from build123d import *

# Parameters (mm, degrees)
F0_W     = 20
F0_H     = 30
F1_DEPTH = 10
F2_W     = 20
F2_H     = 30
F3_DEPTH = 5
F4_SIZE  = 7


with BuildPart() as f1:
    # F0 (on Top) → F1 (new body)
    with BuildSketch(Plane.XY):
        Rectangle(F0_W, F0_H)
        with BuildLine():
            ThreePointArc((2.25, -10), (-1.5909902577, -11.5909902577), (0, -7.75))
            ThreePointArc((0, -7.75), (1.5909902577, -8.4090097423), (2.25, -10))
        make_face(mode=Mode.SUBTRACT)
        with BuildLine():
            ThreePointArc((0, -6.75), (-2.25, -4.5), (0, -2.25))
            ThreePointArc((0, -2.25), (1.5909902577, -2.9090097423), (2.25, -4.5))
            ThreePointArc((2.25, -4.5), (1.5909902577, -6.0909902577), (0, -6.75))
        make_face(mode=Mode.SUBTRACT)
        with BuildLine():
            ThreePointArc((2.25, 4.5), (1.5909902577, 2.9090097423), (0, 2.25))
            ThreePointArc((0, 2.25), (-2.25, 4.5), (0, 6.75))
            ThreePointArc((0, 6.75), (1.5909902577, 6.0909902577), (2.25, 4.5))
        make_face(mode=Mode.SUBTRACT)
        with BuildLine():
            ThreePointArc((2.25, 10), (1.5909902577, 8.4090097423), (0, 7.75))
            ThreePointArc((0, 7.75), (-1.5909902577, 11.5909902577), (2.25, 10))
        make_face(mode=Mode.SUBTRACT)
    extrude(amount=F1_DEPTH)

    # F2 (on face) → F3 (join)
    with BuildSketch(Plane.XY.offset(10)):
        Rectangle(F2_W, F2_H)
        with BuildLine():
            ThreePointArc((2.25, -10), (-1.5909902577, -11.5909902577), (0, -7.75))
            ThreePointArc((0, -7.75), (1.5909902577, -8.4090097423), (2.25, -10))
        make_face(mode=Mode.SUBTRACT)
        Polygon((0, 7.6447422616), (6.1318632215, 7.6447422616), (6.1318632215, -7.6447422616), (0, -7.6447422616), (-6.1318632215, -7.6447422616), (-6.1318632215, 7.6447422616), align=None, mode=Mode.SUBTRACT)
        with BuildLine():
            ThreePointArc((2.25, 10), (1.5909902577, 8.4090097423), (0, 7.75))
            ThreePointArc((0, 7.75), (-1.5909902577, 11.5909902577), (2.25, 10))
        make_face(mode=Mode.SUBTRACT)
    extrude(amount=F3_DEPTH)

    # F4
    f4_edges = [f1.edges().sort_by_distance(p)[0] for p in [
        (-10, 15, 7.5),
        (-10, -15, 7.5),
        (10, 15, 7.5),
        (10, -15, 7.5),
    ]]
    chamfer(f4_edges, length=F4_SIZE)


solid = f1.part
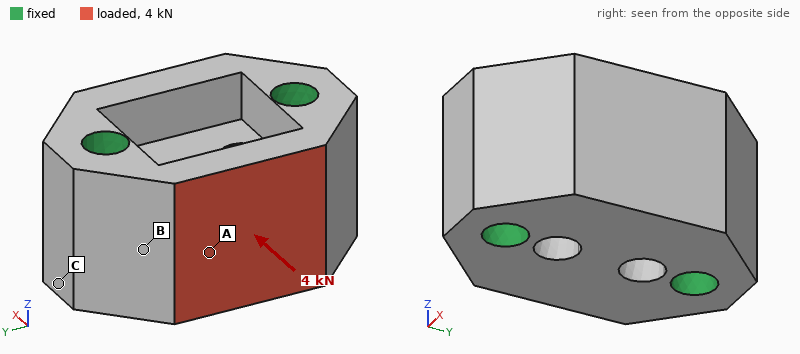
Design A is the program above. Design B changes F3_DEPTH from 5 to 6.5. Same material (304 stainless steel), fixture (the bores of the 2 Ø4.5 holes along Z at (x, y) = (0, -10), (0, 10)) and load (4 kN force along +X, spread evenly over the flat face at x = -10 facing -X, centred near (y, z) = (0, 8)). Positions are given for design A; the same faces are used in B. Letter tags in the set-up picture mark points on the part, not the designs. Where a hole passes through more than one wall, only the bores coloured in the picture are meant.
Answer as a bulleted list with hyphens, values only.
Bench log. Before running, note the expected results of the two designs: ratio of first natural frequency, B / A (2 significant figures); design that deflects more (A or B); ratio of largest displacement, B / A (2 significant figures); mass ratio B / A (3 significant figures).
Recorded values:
- 0.99
- B
- 1.2
- 1.07
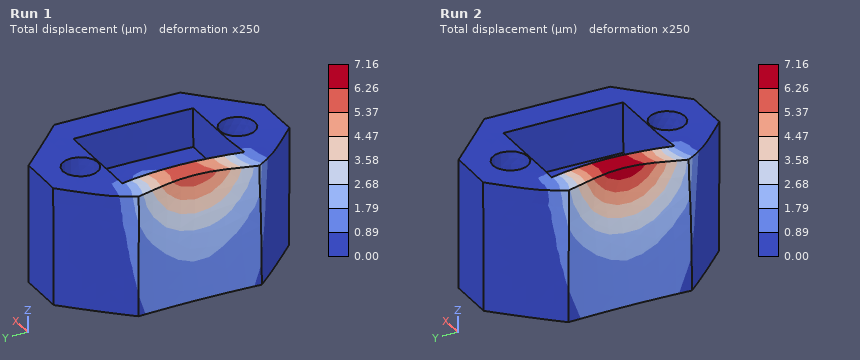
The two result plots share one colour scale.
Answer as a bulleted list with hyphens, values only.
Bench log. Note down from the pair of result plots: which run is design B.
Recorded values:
- Run 2
